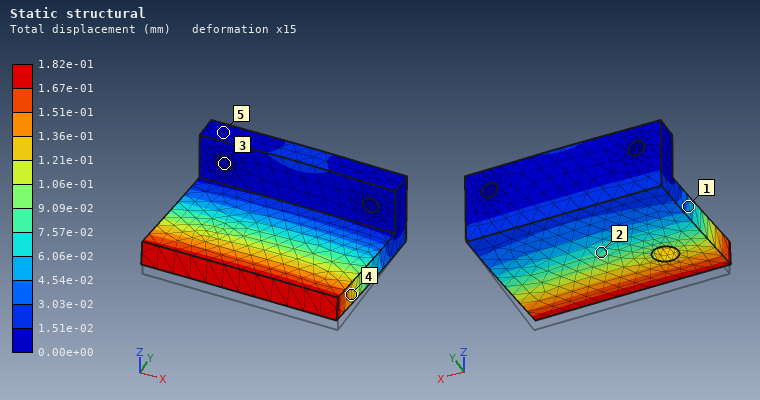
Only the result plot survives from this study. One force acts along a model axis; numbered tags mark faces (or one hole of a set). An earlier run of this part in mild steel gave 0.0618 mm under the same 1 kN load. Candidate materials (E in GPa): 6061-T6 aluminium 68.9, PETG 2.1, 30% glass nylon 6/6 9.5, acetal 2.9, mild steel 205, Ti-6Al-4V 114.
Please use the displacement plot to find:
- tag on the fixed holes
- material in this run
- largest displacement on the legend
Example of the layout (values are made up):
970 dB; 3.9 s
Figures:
3; 6061-T6 aluminium; 1.82e-01 mm
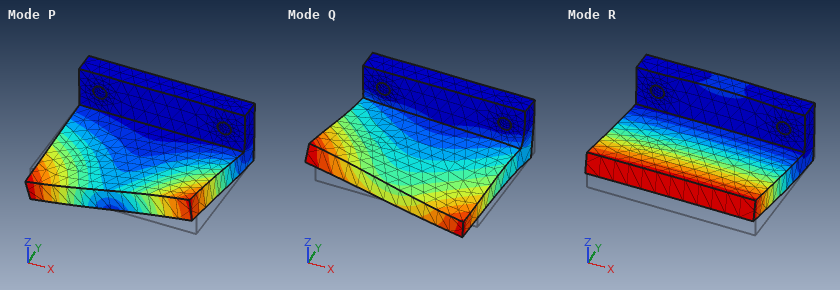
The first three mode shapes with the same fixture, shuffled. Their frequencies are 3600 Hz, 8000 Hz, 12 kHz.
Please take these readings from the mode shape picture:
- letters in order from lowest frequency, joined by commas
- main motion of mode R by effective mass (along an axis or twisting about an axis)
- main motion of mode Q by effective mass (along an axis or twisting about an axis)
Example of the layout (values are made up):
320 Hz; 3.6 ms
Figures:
R, P, Q; along Z; along X
